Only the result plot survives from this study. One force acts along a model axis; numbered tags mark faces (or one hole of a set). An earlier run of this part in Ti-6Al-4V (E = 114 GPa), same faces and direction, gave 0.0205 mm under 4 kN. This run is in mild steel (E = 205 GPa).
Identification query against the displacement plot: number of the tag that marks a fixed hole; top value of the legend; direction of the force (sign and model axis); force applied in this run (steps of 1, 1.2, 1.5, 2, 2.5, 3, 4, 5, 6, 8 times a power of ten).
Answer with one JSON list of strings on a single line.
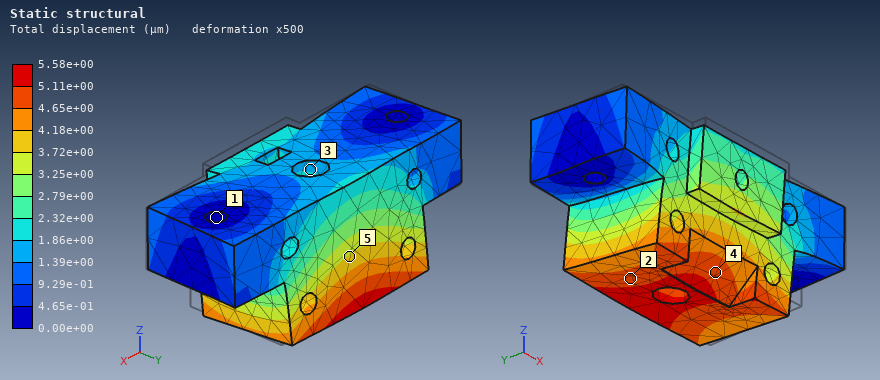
["1", "5.58e+00 µm", "+Y", "2 kN"]
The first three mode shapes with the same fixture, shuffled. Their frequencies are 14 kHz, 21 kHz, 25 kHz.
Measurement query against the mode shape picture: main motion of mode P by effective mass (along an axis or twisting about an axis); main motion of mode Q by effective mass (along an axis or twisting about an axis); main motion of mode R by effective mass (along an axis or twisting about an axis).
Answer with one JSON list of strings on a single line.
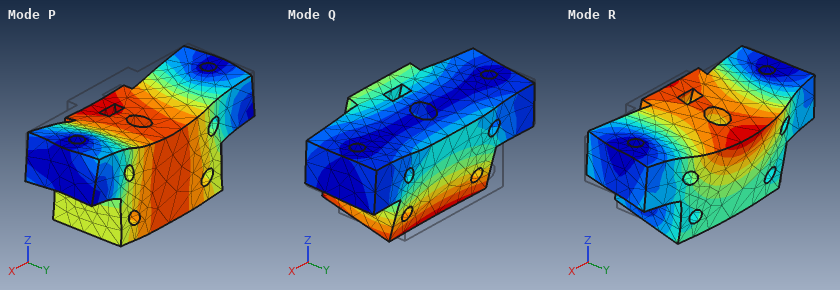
["along Z", "along Y", "along Y"]
